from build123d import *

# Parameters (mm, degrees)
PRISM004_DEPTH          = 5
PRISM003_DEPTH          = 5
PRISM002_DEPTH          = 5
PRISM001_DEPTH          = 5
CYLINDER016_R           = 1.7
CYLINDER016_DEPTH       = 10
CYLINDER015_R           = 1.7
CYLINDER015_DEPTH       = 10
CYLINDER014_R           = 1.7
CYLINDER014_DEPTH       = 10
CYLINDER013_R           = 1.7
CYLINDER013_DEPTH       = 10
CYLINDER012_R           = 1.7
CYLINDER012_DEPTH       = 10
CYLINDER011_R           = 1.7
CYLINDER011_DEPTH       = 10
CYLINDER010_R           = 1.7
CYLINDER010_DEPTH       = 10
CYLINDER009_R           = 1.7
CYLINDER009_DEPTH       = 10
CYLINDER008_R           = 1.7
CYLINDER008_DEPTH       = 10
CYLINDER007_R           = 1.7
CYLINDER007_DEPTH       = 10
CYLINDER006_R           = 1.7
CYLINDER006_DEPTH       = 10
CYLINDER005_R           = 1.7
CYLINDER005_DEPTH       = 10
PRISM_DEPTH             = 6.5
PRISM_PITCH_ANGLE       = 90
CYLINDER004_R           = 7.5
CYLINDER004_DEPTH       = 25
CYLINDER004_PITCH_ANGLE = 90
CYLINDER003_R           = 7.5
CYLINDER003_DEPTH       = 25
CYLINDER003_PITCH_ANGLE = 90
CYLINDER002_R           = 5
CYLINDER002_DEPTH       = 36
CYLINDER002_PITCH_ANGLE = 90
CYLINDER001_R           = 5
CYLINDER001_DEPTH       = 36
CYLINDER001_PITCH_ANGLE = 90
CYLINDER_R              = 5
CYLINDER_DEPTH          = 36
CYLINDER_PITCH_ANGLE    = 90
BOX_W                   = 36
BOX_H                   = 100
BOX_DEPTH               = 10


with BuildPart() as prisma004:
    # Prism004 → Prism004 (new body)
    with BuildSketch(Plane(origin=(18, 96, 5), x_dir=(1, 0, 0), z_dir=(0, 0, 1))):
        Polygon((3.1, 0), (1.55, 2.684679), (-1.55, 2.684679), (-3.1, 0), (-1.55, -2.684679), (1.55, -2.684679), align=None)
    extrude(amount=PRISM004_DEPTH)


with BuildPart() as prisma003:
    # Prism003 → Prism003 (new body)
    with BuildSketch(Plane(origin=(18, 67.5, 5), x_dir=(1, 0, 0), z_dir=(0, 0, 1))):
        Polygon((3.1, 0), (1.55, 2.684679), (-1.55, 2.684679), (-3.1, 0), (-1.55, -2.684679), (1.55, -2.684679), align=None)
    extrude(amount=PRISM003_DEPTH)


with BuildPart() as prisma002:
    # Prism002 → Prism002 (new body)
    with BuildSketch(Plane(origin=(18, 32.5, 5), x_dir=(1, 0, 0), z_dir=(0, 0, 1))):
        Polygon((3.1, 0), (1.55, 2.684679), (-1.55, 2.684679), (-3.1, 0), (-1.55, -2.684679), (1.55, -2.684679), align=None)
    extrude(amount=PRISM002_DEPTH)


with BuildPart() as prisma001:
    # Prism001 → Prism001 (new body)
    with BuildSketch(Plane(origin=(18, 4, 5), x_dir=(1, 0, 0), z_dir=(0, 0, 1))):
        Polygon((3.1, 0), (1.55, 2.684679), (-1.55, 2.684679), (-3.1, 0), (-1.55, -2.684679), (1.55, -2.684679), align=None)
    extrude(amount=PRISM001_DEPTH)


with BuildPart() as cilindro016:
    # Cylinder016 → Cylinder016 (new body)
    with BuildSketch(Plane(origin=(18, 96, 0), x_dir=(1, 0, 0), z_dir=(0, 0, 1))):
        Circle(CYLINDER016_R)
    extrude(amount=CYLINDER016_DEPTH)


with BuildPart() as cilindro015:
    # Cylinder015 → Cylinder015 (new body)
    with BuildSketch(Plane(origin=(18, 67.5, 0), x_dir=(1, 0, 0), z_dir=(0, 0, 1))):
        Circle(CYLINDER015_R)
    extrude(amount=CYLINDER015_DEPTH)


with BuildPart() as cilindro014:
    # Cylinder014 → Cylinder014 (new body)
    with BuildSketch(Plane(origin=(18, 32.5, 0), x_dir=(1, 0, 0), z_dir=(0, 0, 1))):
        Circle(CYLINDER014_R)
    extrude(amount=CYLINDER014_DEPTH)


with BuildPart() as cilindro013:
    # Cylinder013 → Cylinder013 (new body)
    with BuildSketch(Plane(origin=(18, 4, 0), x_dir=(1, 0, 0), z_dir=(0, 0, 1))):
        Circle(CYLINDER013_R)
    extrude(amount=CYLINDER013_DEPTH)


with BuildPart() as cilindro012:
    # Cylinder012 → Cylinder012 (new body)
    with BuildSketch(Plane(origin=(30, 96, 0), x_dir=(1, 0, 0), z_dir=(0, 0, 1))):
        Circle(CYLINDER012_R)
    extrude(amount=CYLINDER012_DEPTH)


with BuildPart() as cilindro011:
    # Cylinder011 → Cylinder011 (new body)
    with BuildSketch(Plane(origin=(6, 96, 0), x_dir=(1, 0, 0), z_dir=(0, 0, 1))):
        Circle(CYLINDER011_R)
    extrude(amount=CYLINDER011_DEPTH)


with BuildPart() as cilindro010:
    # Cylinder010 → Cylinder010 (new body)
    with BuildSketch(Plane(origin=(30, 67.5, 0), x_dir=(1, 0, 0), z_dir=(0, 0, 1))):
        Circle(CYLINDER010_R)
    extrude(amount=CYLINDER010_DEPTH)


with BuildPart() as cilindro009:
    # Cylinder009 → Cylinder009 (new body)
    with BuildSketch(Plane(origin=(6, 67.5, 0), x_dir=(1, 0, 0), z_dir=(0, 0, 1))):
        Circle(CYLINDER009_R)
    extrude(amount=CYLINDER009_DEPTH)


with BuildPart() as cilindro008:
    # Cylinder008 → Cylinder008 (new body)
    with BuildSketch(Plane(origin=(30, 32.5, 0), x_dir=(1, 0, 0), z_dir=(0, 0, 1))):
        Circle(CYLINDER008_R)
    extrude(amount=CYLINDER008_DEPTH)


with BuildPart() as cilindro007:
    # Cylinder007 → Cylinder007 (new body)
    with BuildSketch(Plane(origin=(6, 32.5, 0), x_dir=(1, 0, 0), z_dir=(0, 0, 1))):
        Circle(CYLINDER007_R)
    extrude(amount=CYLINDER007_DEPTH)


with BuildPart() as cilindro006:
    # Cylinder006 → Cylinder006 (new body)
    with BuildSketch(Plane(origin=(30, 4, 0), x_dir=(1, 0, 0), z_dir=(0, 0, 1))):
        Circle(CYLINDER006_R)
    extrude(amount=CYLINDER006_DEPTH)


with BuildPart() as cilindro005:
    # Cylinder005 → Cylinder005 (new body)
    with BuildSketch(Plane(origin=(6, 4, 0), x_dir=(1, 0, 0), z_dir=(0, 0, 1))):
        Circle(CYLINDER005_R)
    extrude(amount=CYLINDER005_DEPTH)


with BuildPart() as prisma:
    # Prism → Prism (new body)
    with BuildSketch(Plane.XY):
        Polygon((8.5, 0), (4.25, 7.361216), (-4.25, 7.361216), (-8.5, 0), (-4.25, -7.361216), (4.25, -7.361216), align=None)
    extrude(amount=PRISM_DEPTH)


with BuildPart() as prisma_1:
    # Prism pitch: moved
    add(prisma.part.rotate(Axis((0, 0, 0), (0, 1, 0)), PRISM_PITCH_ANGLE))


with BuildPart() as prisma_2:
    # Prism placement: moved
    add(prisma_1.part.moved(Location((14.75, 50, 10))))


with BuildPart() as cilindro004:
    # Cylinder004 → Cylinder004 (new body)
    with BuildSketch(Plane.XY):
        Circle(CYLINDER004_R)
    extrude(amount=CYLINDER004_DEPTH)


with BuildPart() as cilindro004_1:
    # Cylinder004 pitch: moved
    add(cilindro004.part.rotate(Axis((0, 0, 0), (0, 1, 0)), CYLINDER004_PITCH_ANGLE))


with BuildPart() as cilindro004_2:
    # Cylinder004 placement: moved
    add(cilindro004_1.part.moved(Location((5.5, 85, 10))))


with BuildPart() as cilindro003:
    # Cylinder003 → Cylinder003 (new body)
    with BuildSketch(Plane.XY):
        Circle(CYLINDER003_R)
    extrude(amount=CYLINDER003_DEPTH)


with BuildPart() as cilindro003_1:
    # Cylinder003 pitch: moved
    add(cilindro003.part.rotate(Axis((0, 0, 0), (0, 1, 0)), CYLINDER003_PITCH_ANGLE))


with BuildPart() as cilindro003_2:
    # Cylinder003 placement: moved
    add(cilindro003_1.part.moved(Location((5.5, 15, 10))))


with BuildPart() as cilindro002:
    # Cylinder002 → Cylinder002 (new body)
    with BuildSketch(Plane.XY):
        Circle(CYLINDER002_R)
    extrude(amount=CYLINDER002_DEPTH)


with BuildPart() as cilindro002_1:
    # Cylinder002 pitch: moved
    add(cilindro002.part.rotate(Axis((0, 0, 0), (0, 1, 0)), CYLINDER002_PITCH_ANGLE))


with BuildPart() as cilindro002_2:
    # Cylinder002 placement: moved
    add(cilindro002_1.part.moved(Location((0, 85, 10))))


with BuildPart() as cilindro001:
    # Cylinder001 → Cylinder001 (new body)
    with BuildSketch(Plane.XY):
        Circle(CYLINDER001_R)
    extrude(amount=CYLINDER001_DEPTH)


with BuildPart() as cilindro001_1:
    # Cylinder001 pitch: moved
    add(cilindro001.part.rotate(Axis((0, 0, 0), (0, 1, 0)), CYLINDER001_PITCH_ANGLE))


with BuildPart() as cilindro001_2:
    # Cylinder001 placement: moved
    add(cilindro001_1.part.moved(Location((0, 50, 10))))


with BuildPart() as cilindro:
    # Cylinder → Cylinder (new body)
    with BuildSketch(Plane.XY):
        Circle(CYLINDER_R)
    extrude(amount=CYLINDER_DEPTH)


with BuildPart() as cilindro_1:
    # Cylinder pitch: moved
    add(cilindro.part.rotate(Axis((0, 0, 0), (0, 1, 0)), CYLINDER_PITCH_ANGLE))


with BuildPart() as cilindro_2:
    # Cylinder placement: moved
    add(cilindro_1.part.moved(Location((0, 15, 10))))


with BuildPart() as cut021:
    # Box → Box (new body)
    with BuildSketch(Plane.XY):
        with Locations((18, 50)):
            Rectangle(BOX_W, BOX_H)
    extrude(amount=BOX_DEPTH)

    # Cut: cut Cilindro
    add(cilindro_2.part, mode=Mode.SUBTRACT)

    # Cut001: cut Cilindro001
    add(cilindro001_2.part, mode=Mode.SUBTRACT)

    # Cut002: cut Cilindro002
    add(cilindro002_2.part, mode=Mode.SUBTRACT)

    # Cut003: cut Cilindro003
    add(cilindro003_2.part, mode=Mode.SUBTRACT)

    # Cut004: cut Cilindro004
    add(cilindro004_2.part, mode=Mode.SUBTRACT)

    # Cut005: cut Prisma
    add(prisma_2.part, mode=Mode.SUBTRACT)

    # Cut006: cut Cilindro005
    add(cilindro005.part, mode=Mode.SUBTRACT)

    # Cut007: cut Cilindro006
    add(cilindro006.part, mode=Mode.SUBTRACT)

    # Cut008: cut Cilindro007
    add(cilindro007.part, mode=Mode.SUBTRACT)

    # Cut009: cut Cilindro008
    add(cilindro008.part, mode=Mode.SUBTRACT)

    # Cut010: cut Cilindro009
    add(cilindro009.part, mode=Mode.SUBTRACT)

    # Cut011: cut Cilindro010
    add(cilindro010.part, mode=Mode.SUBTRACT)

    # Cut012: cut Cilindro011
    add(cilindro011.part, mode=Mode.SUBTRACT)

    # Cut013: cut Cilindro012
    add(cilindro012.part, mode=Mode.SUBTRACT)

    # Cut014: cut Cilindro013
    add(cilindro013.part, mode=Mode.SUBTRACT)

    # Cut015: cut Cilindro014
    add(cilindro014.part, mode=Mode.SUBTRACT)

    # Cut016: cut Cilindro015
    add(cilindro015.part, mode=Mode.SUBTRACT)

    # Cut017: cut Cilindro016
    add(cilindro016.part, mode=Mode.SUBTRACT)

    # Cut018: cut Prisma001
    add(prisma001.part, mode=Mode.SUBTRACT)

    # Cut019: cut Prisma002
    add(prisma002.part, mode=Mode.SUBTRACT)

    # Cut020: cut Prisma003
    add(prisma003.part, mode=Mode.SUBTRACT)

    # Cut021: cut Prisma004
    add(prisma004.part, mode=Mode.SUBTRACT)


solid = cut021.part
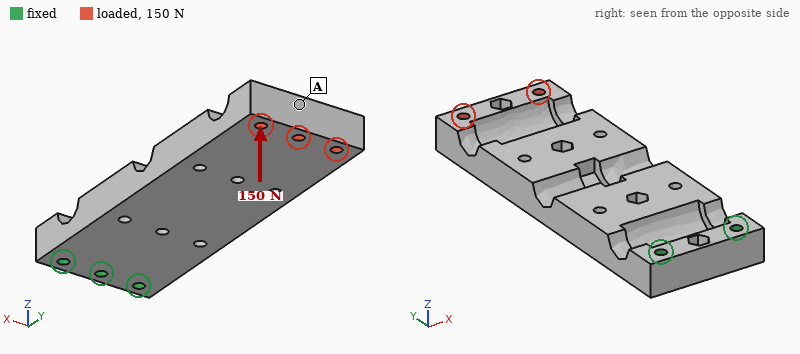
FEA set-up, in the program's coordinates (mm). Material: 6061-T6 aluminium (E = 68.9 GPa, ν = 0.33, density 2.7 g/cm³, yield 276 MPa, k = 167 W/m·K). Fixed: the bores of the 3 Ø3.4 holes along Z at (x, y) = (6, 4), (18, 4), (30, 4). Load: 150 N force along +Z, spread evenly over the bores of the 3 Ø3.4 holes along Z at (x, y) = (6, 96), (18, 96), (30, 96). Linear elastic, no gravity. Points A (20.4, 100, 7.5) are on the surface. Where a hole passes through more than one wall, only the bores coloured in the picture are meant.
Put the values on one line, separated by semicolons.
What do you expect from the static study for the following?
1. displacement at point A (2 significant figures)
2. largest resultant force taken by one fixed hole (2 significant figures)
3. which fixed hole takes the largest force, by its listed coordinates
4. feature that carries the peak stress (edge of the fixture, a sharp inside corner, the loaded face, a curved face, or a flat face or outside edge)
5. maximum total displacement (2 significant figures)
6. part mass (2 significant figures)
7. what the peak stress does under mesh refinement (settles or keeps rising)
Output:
1.0 mm; 790 N; (18, 4); a sharp inside corner; 1.0 mm; 74 g; keeps rising
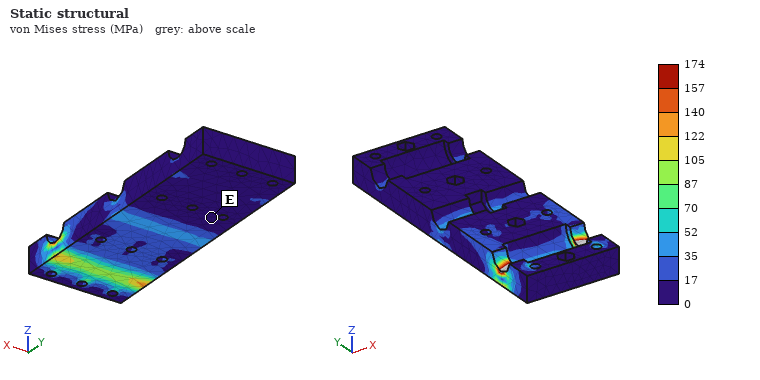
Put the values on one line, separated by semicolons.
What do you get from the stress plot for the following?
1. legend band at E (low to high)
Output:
0 to 17 MPa
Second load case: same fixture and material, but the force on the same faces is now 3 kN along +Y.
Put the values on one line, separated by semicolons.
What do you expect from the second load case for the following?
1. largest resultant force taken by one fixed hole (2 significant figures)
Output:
1.4 kN
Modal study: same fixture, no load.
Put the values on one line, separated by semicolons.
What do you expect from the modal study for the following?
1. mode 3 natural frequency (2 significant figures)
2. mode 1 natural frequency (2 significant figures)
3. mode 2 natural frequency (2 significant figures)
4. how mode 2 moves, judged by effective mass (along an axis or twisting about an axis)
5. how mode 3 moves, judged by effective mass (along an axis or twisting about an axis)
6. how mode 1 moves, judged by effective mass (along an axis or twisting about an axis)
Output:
3200 Hz; 440 Hz; 2400 Hz; along X; along Z; along Z
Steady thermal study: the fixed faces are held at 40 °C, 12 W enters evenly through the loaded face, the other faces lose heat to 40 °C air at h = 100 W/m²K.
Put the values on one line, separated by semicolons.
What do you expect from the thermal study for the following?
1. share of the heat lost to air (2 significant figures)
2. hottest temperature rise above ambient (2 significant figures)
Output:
65 %; 17 K
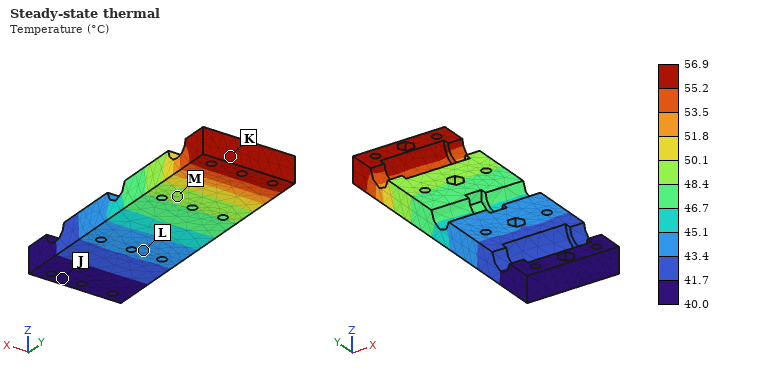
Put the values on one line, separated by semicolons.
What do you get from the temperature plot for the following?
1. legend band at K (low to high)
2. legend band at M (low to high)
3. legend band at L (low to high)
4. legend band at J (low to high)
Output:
55.2 to 56.9 °C; 48.4 to 50.1 °C; 43.4 to 45.1 °C; 40.0 to 41.7 °C
